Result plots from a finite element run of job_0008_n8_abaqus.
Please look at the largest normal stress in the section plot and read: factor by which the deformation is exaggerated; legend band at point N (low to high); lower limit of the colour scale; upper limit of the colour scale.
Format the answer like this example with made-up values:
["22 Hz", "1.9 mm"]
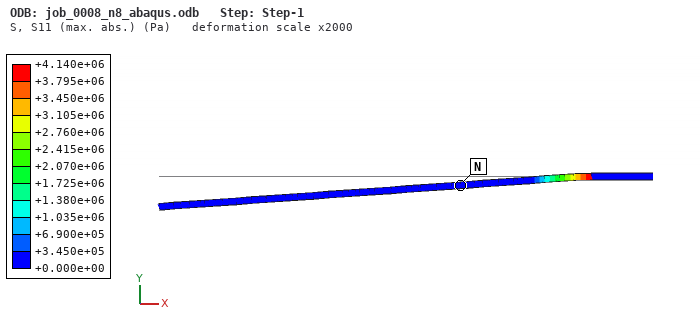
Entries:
["2000", "+0.000e+00 to +3.450e+05 Pa", "+0.000e+00 Pa", "+4.140e+06 Pa"]
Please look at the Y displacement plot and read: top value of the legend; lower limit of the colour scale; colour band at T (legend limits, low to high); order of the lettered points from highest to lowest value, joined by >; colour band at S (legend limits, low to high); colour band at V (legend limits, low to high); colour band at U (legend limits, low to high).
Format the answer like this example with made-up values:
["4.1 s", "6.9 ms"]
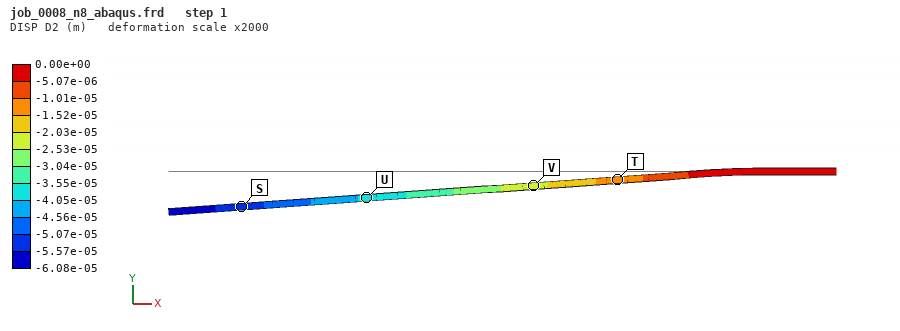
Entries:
["0.00e+00 m", "-6.08e-05 m", "-1.52e-05 to -1.01e-05 m", "T > V > U > S", "-5.57e-05 to -5.07e-05 m", "-2.53e-05 to -2.03e-05 m", "-4.05e-05 to -3.55e-05 m"]
